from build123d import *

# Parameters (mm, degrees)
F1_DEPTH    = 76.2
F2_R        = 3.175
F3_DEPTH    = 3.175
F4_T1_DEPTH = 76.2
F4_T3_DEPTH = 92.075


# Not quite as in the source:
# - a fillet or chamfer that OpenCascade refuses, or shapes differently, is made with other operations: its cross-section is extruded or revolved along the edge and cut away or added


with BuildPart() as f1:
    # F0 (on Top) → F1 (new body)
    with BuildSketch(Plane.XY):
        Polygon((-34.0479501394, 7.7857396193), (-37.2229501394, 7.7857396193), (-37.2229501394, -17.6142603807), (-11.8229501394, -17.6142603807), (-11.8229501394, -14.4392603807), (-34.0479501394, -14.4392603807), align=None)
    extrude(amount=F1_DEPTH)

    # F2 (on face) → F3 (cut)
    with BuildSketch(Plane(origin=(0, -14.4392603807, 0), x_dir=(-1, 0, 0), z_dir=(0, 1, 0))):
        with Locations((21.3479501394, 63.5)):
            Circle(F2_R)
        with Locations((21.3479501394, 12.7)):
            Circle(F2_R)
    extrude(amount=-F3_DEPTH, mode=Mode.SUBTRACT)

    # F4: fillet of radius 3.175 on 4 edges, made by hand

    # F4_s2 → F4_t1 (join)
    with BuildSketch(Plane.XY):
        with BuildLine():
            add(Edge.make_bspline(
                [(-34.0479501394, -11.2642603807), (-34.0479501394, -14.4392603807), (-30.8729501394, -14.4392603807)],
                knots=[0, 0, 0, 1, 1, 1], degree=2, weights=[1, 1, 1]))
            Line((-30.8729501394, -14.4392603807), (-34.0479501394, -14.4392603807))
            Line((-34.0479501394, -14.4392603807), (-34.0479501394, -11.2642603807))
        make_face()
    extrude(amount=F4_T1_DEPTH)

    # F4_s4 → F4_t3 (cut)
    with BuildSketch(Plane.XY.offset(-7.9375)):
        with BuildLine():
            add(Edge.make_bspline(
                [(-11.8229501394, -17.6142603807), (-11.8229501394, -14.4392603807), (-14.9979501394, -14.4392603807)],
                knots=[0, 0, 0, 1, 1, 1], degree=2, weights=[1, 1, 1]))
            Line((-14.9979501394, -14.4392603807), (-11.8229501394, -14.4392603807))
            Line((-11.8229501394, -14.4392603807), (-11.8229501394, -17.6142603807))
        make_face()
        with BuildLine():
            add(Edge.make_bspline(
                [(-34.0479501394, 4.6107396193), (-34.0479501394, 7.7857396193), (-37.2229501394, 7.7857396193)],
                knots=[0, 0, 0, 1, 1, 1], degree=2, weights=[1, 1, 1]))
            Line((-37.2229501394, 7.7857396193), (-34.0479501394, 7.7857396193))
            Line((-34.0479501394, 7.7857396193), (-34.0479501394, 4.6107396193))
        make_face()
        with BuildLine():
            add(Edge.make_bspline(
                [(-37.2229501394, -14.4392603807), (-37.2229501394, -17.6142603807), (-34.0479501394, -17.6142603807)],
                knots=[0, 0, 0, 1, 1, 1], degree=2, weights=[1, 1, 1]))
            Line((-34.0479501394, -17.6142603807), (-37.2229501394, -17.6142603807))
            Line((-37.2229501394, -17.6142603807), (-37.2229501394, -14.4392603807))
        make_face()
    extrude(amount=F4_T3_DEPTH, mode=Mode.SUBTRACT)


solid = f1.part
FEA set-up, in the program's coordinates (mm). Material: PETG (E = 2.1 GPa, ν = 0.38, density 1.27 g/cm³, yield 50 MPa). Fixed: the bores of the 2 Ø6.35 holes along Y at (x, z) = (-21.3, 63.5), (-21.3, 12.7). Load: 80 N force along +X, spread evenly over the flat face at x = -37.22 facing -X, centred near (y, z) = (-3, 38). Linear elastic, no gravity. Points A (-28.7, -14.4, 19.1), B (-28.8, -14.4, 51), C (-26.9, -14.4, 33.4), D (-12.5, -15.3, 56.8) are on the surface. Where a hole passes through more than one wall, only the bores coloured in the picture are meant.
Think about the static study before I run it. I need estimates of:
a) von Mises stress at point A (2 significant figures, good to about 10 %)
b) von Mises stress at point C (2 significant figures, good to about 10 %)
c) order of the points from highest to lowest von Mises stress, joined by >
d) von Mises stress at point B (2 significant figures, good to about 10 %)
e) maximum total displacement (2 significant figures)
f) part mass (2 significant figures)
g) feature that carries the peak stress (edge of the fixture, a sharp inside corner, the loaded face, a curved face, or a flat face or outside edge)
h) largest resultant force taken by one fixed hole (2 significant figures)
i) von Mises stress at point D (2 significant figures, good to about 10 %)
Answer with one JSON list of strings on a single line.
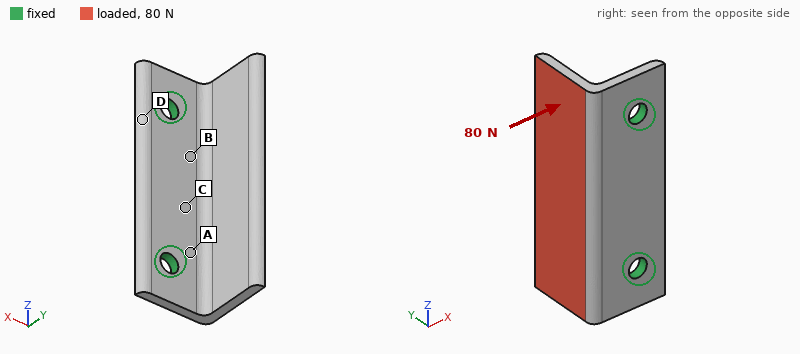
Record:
["8.1 MPa", "4.6 MPa", "A > B > C > D", "6.3 MPa", "0.96 mm", "14 g", "a flat face or outside edge", "41 N", "2.5 MPa"]
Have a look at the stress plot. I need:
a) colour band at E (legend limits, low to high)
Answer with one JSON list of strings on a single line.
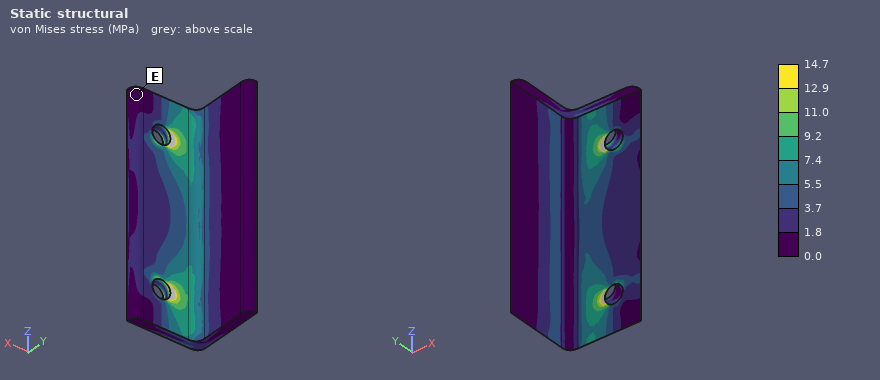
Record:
["0.0 to 1.8 MPa"]
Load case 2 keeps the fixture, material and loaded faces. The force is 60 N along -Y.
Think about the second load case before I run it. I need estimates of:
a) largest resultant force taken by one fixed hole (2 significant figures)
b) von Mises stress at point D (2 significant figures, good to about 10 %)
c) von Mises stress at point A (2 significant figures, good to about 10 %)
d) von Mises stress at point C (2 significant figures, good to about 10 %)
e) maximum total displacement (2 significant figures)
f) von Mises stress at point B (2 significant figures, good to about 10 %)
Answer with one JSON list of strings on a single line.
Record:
["30 N", "1.5 MPa", "4.0 MPa", "1.7 MPa", "0.47 mm", "2.6 MPa"]
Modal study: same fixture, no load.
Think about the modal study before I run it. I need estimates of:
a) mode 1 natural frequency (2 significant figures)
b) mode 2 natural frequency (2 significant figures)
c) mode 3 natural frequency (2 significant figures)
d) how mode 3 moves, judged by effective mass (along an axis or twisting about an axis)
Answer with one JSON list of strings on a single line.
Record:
["640 Hz", "960 Hz", "1700 Hz", "along Y"]
